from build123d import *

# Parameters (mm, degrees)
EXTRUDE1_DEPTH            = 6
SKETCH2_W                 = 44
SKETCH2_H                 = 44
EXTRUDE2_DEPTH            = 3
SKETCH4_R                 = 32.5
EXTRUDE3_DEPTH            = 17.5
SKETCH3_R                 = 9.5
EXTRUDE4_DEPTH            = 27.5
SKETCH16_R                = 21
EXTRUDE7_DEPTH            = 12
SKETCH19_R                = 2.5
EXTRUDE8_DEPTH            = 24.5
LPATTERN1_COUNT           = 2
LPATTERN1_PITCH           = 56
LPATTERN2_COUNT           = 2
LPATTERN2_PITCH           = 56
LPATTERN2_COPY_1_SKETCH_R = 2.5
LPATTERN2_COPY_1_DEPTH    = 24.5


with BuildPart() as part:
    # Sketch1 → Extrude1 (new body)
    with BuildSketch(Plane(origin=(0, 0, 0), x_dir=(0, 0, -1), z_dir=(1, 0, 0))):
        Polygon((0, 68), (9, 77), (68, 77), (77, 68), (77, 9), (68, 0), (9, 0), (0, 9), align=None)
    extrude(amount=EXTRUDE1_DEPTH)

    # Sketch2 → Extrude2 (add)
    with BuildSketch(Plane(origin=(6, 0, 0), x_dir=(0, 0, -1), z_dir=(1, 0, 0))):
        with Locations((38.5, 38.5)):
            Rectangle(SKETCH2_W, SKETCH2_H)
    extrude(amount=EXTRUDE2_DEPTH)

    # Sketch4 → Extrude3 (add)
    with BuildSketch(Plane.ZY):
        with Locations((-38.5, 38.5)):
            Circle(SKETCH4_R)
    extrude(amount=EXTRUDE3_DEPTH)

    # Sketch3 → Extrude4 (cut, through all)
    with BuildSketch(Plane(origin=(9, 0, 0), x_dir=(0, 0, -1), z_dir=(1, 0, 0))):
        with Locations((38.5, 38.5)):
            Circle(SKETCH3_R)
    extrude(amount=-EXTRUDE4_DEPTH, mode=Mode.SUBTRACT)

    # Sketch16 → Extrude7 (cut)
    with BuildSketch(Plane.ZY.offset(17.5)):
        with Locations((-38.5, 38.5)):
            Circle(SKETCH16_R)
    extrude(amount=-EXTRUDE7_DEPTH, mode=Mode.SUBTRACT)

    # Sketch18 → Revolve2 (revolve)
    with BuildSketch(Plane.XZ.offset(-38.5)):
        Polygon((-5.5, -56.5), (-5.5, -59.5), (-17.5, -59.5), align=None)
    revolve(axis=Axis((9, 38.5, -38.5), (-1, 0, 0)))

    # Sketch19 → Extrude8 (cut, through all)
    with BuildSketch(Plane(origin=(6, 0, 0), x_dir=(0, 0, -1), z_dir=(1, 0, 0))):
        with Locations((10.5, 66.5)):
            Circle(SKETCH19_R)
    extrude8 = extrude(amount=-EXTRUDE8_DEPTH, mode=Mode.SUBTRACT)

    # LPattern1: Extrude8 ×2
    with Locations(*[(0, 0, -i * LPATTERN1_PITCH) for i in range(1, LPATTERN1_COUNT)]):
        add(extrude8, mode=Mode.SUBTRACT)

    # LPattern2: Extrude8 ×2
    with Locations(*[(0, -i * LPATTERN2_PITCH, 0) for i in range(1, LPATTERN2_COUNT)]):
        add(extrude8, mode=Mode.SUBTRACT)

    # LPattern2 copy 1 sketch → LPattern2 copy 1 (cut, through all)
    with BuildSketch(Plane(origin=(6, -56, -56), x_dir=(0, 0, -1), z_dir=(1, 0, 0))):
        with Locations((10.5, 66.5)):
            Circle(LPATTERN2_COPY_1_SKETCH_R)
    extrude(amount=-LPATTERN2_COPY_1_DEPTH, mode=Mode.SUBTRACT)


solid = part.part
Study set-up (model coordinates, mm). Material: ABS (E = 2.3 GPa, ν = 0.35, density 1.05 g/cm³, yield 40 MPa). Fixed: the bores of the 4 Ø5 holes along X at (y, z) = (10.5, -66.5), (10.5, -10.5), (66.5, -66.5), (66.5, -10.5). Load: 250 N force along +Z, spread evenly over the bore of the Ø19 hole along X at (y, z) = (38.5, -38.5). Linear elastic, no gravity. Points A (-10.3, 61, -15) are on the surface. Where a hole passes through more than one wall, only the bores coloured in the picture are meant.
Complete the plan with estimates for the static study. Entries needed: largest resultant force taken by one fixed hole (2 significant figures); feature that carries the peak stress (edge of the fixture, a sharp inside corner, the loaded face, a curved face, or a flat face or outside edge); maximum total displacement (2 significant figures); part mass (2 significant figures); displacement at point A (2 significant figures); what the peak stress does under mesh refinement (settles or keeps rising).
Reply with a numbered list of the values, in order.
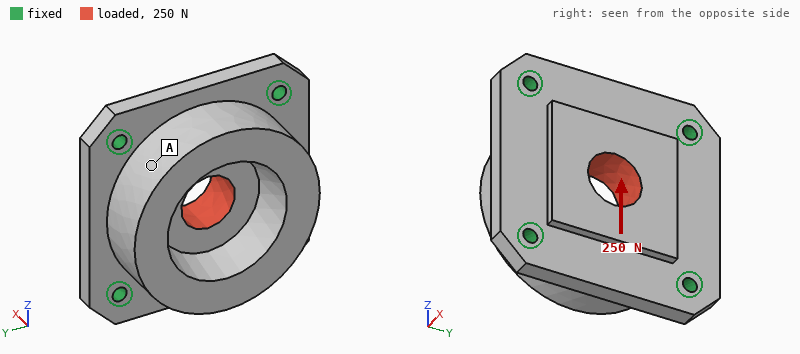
1. 66 N
2. edge of the fixture
3. 7.7 µm
4. 84 g
5. 4.2 µm
6. keeps rising
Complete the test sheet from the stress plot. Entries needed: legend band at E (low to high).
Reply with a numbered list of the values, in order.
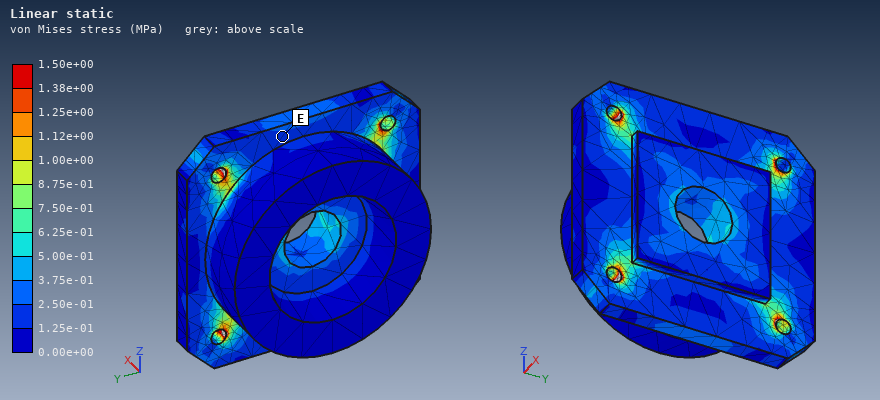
1. 1.25e-01 to 2.50e-01 MPa
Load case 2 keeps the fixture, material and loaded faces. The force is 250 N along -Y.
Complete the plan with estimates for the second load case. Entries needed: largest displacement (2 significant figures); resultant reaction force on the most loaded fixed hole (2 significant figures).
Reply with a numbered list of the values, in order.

1. 7.7 µm
2. 66 N
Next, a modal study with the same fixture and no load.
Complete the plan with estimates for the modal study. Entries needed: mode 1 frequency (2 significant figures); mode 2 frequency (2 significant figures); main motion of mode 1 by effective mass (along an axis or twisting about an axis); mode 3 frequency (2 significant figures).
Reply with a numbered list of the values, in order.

1. 2400 Hz
2. 3000 Hz
3. along X
4. 3000 Hz
